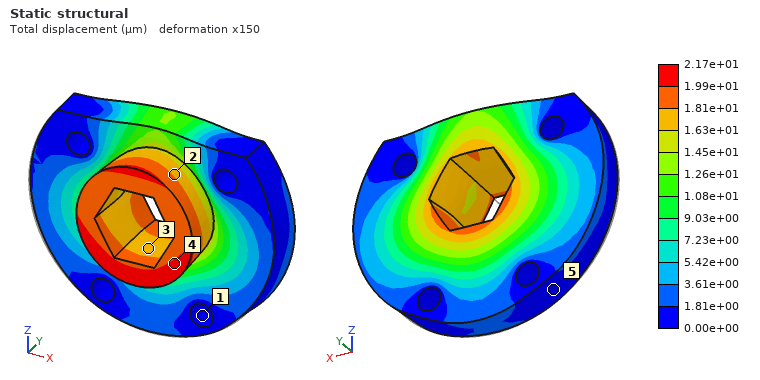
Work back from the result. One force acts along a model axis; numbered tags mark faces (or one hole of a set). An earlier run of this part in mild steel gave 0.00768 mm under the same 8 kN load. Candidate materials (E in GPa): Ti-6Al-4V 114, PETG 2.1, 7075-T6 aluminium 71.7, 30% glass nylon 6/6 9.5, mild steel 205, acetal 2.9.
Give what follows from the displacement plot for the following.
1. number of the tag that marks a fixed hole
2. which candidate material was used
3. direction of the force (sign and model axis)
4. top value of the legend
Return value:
1
7075-T6 aluminium
+Y
2.17e+01 µm
